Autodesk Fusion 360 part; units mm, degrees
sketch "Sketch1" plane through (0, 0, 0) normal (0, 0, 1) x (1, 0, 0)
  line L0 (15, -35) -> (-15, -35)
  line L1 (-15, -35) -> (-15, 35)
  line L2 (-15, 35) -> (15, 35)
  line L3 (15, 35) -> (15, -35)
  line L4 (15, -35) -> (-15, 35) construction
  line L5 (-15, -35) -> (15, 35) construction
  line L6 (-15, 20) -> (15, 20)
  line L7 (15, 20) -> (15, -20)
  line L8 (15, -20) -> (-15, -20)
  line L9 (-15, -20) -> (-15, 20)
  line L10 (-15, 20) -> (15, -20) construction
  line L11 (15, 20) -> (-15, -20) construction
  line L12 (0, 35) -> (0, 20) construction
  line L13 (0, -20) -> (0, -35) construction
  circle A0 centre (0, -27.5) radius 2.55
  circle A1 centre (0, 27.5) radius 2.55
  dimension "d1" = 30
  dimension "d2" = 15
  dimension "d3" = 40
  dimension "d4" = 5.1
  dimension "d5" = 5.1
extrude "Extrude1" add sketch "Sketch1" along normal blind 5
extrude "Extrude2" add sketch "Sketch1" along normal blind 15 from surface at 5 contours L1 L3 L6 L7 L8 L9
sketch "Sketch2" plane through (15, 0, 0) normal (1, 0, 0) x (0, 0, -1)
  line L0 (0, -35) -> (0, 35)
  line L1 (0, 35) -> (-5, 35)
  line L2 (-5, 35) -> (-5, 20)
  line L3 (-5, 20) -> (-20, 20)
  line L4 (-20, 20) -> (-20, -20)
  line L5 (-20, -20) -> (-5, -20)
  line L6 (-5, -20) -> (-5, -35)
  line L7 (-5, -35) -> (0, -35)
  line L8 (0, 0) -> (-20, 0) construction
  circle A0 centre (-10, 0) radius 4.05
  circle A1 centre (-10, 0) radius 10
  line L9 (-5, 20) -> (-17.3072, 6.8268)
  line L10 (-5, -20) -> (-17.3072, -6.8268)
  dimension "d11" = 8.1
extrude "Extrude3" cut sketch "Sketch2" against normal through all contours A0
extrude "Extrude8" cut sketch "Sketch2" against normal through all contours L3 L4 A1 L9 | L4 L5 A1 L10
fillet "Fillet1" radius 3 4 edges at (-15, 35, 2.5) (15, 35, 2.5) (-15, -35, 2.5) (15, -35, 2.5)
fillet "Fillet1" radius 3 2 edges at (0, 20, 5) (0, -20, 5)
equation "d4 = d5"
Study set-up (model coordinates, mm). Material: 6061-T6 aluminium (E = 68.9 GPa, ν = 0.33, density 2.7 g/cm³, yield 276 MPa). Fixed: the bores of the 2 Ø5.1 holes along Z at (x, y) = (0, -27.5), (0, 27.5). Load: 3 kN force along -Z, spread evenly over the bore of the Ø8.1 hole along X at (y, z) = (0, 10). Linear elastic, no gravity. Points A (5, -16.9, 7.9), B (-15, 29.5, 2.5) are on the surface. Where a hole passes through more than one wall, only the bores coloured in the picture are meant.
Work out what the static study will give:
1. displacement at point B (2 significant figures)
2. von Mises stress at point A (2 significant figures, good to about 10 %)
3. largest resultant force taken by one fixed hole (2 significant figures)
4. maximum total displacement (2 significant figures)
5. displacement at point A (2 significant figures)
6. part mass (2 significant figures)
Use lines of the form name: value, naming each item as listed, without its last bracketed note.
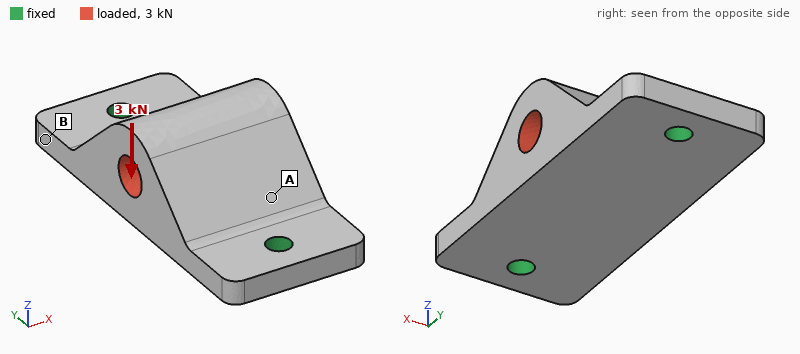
displacement at point B: 6.2 µm
von Mises stress at point A: 36 MPa
largest resultant force taken by one fixed hole: 1.9 kN
maximum total displacement: 27 µm
displacement at point A: 18 µm
part mass: 52 g
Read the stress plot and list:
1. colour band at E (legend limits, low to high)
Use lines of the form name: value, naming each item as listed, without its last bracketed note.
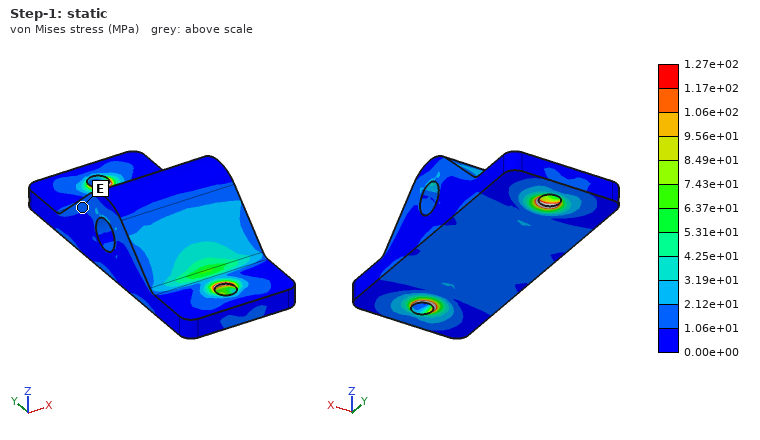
colour band at E: 1.06e+01 to 2.12e+01 MPa
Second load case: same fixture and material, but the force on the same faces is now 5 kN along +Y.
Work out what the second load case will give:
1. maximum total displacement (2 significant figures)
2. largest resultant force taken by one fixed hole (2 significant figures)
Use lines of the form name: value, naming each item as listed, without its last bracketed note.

maximum total displacement: 12 µm
largest resultant force taken by one fixed hole: 2.6 kN
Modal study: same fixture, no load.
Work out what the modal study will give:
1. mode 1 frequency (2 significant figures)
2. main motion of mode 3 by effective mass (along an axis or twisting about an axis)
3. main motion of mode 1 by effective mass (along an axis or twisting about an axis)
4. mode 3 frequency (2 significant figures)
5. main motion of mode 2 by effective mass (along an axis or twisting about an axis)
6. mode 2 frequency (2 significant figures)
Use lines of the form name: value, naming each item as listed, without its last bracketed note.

mode 1 frequency: 5400 Hz
main motion of mode 3 by effective mass: along X
main motion of mode 1 by effective mass: along X
mode 3 frequency: 15 kHz
main motion of mode 2 by effective mass: along Z
mode 2 frequency: 9100 Hz
